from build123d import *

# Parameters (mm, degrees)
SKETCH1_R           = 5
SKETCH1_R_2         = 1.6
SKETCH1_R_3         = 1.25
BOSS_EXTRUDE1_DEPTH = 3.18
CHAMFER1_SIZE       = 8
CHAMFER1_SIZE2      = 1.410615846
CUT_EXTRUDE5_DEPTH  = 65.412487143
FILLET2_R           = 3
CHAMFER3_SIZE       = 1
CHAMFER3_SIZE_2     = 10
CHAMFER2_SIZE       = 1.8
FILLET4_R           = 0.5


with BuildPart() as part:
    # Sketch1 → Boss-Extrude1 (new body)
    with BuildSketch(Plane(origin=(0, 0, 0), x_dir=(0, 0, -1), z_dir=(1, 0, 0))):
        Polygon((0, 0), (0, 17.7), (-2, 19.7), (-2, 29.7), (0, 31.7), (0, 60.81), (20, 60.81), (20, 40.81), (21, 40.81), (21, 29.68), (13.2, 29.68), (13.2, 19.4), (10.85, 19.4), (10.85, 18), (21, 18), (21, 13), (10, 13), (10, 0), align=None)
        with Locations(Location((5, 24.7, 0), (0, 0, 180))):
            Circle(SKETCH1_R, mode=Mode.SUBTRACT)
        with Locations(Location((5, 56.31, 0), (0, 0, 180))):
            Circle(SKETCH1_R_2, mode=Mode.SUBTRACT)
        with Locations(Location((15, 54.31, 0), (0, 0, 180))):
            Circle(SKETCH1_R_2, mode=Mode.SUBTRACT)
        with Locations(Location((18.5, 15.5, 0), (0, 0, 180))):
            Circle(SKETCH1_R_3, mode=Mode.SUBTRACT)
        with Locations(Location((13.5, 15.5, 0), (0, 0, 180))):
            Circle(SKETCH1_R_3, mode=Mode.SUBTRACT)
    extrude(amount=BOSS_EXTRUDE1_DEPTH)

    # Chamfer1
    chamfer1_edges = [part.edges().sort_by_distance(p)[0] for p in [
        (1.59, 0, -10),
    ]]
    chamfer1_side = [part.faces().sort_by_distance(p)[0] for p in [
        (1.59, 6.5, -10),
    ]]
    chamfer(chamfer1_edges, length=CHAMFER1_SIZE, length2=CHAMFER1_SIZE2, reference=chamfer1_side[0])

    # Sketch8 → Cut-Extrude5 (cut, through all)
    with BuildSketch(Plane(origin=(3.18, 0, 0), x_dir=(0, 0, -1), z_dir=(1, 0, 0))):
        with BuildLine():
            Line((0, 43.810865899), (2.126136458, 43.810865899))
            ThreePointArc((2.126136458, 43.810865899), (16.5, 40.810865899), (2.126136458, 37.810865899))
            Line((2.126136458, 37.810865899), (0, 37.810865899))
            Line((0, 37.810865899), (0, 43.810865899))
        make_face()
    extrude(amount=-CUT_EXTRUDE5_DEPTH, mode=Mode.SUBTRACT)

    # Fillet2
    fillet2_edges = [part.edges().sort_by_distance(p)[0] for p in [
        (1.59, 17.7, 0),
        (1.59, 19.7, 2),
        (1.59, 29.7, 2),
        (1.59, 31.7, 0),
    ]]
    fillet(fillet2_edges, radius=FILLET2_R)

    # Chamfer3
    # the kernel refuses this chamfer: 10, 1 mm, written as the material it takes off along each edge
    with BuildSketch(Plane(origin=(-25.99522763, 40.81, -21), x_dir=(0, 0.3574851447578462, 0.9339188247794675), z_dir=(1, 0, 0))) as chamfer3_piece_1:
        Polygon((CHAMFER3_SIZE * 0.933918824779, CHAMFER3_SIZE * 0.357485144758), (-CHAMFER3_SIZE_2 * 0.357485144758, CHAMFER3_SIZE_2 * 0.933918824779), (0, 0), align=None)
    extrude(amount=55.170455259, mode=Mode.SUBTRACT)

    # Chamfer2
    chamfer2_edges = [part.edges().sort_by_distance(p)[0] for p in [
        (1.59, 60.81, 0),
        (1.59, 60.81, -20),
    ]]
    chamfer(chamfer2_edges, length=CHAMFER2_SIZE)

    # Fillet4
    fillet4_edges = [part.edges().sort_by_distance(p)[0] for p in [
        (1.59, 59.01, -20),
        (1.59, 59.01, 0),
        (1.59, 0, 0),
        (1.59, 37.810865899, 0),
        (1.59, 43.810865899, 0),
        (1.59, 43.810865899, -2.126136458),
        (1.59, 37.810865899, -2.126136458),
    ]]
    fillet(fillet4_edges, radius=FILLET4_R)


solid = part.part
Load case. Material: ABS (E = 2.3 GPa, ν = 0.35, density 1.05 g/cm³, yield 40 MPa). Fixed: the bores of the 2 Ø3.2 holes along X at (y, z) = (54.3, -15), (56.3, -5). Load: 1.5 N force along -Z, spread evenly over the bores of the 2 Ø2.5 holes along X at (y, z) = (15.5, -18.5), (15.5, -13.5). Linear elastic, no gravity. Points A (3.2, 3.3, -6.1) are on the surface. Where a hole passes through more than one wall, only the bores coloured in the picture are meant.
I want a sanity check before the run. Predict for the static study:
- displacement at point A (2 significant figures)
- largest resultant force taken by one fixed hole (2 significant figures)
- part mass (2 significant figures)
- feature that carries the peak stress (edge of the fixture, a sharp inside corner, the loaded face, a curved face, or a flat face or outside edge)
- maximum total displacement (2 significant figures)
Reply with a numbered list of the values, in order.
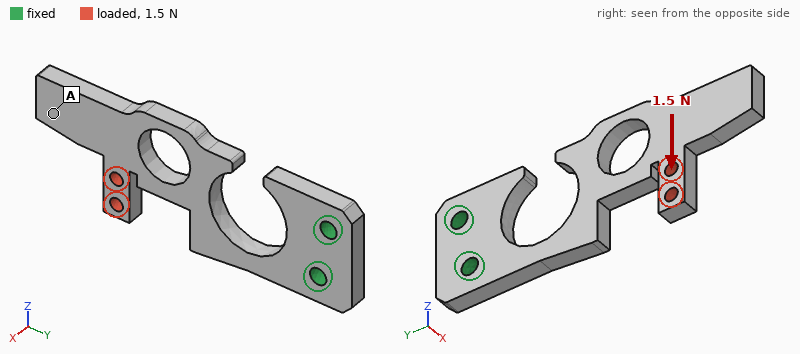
1. 0.59 mm
2. 4.9 N
3. 2.5 g
4. a curved face
5. 0.67 mm
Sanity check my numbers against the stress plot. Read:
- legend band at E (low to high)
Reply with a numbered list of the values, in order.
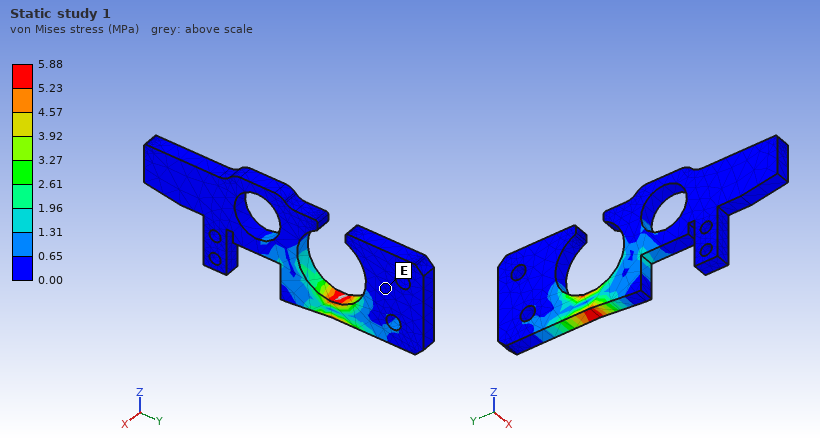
1. 0.00 to 0.65 MPa
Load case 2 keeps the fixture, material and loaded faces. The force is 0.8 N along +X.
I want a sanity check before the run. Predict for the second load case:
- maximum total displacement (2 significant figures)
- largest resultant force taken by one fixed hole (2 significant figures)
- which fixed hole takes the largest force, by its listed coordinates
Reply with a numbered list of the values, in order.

1. 0.75 mm
2. 1.3 N
3. (54.3, -15)
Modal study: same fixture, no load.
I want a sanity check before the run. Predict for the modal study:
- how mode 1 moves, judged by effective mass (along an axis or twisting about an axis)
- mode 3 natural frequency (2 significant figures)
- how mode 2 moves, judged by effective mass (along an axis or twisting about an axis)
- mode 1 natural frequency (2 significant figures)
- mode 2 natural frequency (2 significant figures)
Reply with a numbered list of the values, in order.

1. along X
2. 700 Hz
3. along Z
4. 170 Hz
5. 250 Hz
